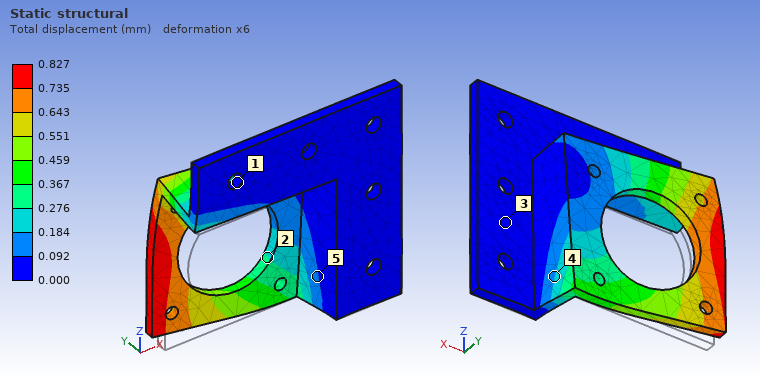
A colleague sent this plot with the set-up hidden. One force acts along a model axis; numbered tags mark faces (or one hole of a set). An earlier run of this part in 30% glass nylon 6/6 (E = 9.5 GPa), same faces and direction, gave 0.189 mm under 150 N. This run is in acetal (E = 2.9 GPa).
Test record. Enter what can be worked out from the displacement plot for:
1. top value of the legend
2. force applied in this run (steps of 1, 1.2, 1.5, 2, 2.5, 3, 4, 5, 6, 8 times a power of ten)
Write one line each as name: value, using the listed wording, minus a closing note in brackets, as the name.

top value of the legend: 0.827 mm
force applied in this run: 200 N
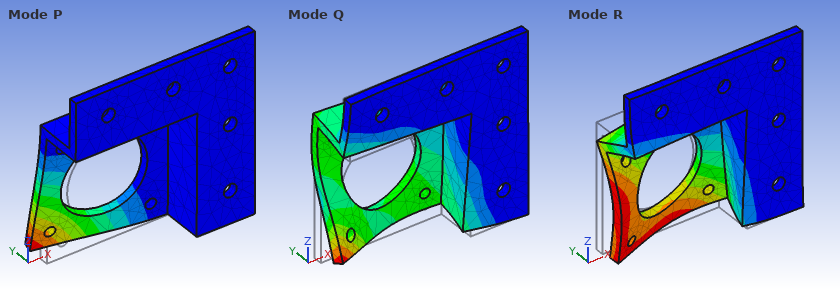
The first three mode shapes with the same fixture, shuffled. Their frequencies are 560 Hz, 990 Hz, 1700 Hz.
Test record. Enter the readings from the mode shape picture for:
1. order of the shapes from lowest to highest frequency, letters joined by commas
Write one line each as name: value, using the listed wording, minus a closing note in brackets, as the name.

order of the shapes from lowest to highest frequency, letters joined by commas: P, R, Q
